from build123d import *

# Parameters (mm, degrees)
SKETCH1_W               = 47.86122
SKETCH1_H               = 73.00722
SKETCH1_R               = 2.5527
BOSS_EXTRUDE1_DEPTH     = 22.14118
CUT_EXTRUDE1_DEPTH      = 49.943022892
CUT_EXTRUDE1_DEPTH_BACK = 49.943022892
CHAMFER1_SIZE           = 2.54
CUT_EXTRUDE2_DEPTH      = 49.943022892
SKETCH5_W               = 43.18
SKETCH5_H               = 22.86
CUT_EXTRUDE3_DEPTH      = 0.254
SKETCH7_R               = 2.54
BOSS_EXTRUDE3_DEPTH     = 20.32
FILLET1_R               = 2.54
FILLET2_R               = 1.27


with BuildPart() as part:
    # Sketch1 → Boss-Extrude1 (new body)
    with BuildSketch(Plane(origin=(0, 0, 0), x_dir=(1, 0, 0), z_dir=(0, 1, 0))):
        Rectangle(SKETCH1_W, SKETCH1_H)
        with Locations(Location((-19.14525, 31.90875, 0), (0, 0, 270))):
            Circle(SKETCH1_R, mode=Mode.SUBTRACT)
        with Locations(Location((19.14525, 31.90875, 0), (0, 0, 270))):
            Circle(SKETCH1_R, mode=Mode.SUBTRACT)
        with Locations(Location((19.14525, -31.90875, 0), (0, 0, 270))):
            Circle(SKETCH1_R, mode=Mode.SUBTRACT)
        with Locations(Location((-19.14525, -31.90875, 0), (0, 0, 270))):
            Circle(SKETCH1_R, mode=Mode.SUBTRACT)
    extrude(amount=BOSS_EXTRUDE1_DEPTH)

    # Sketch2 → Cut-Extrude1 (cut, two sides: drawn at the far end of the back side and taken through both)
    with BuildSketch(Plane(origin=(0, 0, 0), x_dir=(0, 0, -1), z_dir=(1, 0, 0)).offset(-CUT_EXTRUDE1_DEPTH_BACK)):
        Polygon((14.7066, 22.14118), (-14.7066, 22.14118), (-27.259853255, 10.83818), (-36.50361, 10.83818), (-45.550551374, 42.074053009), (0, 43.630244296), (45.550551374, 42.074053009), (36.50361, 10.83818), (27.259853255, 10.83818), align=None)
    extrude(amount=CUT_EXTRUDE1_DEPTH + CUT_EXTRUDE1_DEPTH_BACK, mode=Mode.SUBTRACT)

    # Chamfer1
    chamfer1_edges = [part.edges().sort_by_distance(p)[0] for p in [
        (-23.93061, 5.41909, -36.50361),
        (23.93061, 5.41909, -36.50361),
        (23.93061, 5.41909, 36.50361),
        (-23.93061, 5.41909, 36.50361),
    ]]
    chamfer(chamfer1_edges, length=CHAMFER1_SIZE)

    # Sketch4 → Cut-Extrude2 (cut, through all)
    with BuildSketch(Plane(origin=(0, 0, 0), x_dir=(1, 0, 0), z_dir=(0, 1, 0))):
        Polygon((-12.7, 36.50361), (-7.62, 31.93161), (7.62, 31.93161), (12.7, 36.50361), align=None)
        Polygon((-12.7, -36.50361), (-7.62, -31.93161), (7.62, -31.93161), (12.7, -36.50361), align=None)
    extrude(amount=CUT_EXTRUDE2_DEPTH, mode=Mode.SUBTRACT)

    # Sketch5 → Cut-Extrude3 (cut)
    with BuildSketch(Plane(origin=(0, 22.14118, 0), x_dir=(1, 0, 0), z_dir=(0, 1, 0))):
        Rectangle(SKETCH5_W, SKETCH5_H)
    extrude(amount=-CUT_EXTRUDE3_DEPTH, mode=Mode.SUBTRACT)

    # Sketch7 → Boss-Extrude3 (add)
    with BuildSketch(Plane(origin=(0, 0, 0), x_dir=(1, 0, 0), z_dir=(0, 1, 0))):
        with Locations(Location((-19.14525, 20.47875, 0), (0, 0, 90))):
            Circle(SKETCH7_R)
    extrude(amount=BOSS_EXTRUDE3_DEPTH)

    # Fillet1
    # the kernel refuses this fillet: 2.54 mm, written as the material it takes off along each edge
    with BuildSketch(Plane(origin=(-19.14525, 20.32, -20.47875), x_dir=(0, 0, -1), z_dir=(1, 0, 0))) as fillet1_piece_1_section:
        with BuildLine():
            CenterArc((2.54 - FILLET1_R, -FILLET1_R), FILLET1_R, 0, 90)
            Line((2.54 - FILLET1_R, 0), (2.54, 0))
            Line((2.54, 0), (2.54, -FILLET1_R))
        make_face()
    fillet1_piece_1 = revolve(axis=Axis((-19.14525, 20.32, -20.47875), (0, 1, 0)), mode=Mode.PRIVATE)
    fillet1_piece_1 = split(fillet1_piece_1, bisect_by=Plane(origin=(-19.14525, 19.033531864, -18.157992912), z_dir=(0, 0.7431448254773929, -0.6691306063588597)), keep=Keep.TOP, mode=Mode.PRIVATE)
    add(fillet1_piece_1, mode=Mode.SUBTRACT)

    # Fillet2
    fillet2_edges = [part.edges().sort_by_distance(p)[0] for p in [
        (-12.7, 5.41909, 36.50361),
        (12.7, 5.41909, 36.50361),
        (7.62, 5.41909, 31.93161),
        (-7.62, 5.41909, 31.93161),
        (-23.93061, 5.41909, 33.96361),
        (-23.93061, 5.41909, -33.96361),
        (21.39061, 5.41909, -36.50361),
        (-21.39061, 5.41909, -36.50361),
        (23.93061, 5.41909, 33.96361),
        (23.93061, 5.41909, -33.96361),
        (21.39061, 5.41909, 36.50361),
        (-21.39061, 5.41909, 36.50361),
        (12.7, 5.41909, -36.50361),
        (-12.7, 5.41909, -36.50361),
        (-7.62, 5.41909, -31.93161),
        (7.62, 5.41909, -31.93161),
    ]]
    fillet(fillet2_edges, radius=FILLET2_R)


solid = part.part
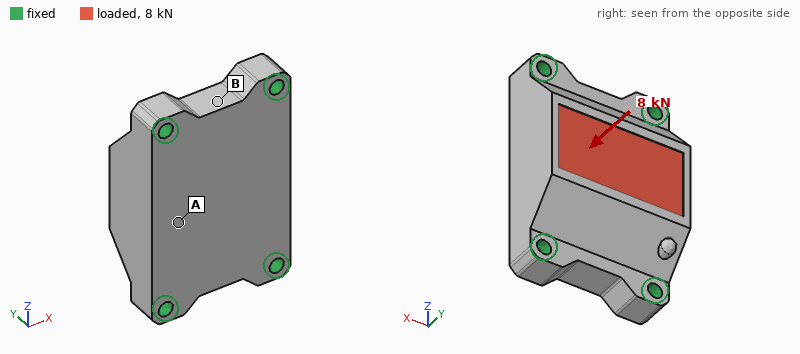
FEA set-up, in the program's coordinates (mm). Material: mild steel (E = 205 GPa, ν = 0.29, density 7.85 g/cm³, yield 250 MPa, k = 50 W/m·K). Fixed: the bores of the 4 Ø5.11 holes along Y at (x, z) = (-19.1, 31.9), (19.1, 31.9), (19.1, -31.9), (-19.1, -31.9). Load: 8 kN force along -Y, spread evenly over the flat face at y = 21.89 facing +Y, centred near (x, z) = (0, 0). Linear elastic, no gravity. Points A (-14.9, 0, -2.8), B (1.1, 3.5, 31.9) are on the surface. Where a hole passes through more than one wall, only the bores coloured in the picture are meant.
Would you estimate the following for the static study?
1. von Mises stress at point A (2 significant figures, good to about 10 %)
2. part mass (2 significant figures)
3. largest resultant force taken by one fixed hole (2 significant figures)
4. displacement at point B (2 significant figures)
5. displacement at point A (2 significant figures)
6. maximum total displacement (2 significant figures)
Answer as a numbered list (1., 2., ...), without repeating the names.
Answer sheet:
1. 15 MPa
2. 450 g
3. 2.4 kN
4. 1.6 µm
5. 4.6 µm
6. 5.0 µm
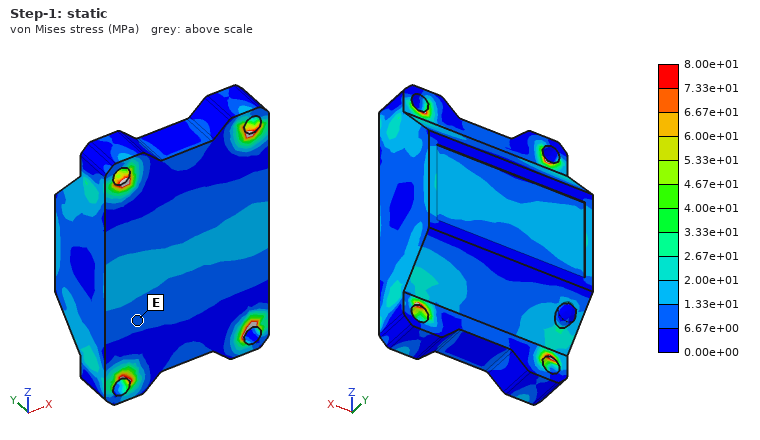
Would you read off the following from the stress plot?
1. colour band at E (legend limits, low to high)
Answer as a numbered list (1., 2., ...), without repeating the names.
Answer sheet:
1. 6.67e+00 to 1.33e+01 MPa
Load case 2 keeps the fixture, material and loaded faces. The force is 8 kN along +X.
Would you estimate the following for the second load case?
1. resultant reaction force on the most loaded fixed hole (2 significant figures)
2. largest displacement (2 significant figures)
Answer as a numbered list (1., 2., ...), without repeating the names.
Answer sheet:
1. 3.2 kN
2. 7.6 µm
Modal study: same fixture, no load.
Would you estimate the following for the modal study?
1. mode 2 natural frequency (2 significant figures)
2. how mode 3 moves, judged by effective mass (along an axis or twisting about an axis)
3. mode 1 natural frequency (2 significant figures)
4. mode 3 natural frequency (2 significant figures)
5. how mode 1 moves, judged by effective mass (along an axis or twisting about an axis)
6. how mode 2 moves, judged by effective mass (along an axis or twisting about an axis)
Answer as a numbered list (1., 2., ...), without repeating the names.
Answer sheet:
1. 14 kHz
2. along X
3. 12 kHz
4. 18 kHz
5. along Y
6. along X
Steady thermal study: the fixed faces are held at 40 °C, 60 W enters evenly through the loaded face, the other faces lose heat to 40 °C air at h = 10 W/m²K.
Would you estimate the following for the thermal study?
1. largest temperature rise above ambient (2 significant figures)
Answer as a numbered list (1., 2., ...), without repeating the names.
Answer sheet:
1. 36 K
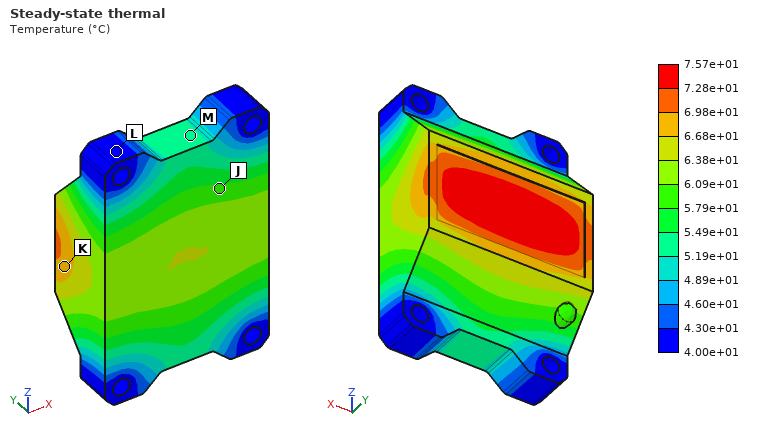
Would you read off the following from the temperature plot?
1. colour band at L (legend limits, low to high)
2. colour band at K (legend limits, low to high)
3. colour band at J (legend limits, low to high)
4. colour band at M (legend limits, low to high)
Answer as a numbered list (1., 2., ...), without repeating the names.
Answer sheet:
1. 4.00e+01 to 4.30e+01 °C
2. 6.68e+01 to 6.98e+01 °C
3. 5.79e+01 to 6.09e+01 °C
4. 5.19e+01 to 5.49e+01 °C
